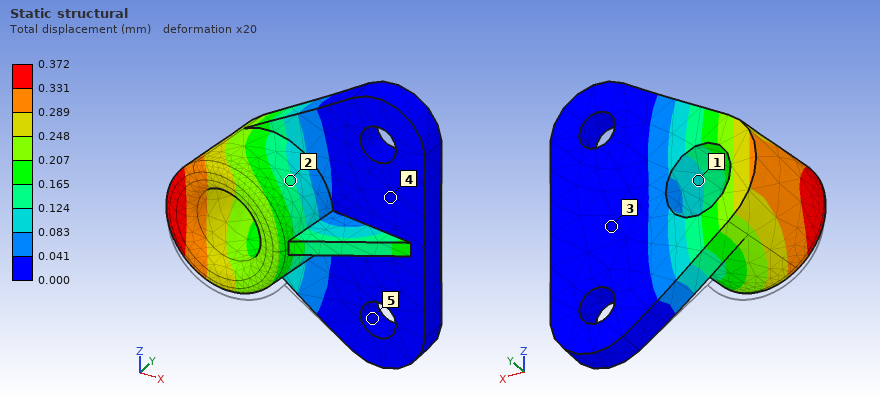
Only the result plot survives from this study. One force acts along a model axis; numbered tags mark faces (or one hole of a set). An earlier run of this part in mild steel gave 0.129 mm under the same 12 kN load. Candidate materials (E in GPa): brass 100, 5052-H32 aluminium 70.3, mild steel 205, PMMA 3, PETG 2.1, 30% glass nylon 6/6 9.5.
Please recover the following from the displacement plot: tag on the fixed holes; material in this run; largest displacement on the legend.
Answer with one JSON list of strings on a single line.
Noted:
["5", "5052-H32 aluminium", "0.372 mm"]
